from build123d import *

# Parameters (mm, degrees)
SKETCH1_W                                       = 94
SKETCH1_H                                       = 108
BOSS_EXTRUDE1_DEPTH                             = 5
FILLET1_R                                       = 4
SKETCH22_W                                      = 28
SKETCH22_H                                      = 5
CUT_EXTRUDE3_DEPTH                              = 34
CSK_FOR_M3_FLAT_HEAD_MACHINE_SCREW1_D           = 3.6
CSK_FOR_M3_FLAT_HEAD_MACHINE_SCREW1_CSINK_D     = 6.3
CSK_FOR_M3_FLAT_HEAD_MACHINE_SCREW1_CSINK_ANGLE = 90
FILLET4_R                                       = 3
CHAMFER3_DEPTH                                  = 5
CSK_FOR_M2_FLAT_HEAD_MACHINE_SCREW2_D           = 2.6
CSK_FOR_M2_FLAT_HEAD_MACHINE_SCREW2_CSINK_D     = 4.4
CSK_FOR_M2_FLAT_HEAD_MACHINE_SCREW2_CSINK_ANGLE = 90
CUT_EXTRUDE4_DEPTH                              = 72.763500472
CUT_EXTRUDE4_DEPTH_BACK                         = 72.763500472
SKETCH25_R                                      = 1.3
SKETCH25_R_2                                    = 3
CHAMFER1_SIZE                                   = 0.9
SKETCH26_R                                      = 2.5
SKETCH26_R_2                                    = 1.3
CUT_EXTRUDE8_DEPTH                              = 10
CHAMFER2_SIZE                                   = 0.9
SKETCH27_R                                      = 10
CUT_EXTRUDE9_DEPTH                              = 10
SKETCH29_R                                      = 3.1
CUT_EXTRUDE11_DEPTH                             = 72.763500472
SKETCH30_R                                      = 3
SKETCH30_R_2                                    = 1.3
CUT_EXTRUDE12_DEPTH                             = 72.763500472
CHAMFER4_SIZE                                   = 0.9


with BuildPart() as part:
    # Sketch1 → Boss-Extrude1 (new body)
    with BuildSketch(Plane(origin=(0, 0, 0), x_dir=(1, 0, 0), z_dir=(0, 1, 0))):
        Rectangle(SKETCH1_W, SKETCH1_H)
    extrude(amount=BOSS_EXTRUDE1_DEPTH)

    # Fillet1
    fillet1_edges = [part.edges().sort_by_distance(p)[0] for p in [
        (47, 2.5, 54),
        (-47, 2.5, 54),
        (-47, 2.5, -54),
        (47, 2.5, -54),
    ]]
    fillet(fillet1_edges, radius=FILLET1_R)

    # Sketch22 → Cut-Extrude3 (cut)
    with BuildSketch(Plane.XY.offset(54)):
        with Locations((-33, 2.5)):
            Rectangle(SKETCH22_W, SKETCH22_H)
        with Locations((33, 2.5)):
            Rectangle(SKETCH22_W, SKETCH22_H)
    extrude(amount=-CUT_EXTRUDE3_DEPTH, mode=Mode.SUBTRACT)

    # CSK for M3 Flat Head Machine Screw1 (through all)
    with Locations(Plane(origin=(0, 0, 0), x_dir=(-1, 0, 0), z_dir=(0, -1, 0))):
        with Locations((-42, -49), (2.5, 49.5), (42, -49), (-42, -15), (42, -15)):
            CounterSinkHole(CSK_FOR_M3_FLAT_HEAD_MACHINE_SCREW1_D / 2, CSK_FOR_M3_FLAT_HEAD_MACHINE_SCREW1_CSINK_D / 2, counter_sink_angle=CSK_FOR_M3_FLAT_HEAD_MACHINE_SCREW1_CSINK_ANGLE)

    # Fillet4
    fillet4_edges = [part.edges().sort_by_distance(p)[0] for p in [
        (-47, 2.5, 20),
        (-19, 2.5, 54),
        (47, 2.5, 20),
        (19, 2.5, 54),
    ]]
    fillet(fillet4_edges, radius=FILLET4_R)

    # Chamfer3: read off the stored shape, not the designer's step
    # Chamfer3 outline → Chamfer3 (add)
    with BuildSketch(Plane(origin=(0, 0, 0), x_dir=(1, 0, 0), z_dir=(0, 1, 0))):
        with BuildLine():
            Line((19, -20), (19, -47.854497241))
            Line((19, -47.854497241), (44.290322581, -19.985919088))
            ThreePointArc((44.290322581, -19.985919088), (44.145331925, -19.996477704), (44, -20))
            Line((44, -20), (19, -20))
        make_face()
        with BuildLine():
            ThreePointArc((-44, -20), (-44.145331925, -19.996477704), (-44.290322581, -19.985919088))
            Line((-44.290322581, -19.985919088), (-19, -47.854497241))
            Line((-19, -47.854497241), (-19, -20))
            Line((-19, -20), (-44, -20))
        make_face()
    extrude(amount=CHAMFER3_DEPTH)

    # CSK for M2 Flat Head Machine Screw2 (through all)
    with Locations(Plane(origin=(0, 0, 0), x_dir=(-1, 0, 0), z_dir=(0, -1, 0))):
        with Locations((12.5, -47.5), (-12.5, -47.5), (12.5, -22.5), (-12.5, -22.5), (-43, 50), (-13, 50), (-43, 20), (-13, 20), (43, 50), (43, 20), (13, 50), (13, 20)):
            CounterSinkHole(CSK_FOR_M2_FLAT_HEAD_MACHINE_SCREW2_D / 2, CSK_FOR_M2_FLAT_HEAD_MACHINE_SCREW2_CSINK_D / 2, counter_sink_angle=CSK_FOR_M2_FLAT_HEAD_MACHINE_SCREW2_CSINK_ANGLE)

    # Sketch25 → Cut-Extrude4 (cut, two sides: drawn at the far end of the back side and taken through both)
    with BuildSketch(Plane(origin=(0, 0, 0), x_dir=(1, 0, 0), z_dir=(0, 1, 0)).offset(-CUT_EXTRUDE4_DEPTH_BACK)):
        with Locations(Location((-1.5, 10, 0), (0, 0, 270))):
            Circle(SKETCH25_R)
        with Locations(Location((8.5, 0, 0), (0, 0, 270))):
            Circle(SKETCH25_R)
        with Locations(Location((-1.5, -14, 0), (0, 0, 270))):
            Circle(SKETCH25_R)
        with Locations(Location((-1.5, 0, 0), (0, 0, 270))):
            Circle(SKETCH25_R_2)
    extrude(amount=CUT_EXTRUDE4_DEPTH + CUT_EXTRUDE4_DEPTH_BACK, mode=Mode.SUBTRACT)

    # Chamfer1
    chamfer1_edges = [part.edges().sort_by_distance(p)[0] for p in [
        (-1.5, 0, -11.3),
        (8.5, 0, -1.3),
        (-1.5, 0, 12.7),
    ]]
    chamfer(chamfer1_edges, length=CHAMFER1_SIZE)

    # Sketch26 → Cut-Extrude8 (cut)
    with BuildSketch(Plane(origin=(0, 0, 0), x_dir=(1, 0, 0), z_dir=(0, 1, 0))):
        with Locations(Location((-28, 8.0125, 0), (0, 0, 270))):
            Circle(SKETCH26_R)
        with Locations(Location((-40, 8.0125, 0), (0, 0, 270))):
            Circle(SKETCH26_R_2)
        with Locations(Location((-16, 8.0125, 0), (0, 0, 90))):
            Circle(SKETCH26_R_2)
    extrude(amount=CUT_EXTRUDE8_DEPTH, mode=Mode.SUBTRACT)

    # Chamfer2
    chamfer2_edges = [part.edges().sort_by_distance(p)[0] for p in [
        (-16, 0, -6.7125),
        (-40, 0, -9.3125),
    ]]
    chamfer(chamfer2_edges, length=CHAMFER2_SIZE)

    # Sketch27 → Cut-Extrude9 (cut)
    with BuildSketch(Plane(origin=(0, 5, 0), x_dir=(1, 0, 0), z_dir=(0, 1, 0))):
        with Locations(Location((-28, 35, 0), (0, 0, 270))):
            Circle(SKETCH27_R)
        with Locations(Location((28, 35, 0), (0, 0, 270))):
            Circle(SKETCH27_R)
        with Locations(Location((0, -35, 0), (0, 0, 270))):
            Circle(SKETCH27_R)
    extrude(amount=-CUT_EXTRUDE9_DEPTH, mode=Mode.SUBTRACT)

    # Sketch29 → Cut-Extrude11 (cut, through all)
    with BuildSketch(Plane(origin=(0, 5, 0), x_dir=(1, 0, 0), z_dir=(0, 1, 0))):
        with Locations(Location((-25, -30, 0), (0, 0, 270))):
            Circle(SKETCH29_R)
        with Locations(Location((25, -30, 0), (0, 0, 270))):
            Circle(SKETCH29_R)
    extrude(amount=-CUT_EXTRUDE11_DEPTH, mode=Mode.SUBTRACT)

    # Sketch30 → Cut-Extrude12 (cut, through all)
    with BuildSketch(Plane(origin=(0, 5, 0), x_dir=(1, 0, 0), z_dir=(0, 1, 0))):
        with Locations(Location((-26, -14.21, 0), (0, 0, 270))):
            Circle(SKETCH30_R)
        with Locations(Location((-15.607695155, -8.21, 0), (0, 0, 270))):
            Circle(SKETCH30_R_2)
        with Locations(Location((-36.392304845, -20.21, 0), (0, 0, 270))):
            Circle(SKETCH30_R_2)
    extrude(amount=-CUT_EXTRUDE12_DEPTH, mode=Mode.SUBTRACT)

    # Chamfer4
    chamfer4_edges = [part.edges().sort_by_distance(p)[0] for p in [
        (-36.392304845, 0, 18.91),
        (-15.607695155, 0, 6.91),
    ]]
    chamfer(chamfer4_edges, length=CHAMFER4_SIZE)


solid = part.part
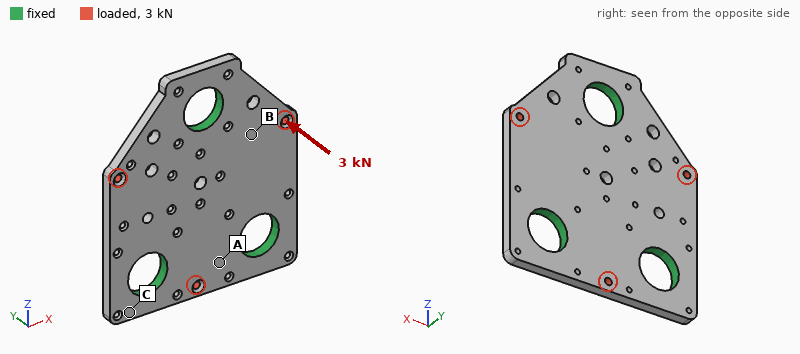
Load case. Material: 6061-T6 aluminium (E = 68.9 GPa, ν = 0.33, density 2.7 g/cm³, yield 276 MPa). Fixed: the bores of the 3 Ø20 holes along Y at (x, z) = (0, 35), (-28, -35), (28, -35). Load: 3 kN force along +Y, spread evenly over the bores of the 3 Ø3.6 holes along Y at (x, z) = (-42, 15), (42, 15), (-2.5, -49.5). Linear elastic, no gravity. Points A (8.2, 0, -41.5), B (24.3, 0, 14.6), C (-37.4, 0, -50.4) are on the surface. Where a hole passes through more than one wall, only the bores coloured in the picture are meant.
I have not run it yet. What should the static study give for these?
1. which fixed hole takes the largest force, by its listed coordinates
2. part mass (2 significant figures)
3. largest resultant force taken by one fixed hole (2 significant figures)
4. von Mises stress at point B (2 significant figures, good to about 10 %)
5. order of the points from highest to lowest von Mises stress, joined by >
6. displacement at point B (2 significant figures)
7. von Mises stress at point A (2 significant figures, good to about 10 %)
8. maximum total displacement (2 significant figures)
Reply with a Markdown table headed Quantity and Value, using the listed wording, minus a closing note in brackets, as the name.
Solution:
| Quantity | Value |
|---|---|
| which fixed hole takes the largest force, by its listed coordinates | (0, 35) |
| part mass | 100 g |
| largest resultant force taken by one fixed hole | 1.2 kN |
| von Mises stress at point B | 68 MPa |
| order of the points from highest to lowest von Mises stress, joined by > | B > A > C |
| displacement at point B | 0.089 mm |
| von Mises stress at point A | 33 MPa |
| maximum total displacement | 0.36 mm |
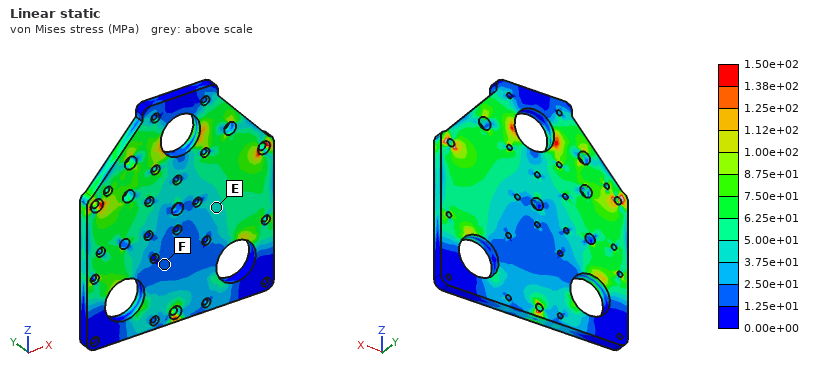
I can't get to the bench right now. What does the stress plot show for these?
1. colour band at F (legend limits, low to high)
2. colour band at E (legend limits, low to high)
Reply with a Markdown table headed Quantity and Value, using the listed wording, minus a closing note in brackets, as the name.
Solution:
| Quantity | Value |
|---|---|
| colour band at F | 1.25e+01 to 2.50e+01 MPa |
| colour band at E | 3.75e+01 to 5.00e+01 MPa |
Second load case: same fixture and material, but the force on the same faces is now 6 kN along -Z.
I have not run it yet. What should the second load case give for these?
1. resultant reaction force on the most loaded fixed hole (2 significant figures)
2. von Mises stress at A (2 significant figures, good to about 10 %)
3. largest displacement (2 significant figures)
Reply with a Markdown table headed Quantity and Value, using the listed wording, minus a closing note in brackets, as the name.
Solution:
| Quantity | Value |
|---|---|
| resultant reaction force on the most loaded fixed hole | 2.5 kN |
| von Mises stress at A | 11 MPa |
| largest displacement | 18 µm |
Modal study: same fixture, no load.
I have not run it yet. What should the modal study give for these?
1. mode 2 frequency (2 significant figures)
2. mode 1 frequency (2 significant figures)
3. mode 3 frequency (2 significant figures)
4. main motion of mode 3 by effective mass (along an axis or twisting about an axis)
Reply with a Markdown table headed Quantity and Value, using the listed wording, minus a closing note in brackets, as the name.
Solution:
| Quantity | Value |
|---|---|
| mode 2 frequency | 4400 Hz |
| mode 1 frequency | 4300 Hz |
| mode 3 frequency | 8100 Hz |
| main motion of mode 3 by effective mass | along Y |
